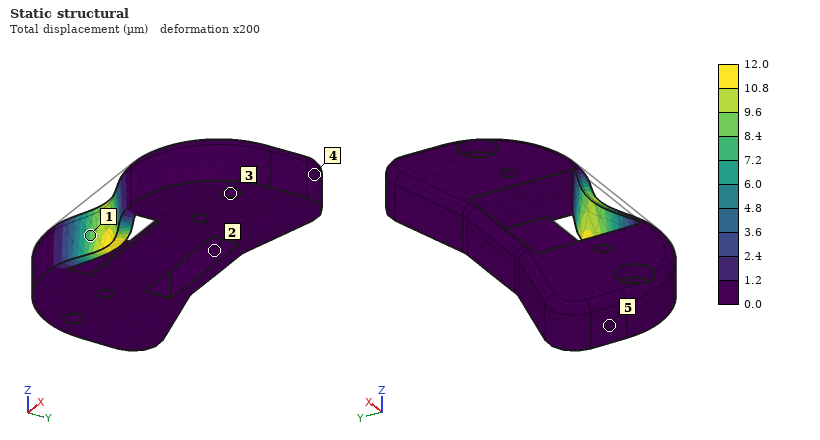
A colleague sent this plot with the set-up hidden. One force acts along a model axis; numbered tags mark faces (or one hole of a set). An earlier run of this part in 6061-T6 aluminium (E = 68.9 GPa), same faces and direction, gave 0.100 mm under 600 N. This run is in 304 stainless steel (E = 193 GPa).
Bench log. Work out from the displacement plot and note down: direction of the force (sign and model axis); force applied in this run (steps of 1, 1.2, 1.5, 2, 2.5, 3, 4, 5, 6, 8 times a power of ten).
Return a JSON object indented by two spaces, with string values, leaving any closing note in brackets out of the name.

{
  "direction of the force": "+Y",
  "force applied in this run": "200 N"
}
